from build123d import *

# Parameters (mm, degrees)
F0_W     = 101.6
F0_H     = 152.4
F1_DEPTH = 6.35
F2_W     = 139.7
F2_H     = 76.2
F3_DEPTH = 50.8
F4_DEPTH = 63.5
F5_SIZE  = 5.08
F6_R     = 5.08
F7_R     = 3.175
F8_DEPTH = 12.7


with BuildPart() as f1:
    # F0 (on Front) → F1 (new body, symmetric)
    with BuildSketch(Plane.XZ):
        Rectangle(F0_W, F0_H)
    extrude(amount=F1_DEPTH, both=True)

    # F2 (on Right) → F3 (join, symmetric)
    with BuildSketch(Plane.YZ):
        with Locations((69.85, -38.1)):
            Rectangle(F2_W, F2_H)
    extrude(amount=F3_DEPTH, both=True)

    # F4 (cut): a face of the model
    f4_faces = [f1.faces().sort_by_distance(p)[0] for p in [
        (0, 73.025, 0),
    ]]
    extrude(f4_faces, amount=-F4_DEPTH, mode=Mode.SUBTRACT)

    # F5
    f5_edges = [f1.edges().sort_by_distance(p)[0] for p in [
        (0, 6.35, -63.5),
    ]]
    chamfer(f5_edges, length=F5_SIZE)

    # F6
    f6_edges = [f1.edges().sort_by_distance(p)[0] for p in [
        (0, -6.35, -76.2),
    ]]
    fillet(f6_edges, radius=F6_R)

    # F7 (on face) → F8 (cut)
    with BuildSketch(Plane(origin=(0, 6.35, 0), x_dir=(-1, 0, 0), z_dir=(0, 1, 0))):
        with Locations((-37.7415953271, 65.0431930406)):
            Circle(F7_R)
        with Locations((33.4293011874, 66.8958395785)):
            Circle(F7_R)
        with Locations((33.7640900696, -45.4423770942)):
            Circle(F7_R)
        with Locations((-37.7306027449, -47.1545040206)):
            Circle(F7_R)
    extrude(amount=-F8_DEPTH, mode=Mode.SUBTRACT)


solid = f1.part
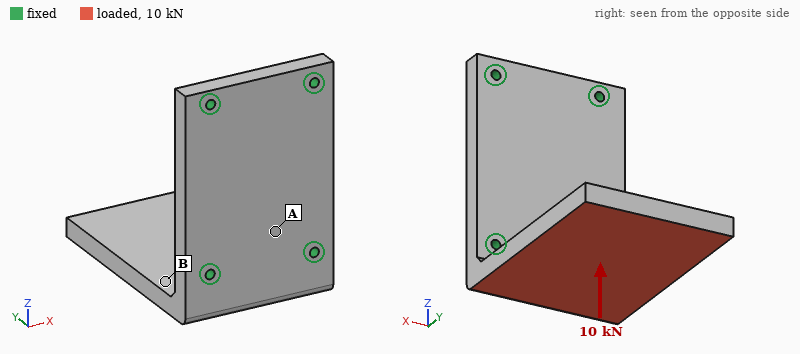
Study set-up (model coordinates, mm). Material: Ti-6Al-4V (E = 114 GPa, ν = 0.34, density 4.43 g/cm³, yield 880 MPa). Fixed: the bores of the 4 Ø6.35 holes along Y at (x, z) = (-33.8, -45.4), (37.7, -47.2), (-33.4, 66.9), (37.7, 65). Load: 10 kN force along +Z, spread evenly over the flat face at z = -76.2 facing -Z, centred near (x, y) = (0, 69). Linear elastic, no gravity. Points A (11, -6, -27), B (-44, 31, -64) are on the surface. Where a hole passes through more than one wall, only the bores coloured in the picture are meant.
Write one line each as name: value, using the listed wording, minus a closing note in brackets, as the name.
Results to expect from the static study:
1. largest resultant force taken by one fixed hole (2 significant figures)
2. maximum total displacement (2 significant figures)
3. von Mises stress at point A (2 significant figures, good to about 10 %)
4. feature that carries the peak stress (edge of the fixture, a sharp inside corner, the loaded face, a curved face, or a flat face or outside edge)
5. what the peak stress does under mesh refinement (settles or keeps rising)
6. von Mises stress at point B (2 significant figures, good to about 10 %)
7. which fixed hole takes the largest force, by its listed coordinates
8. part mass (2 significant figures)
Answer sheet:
largest resultant force taken by one fixed hole: 4.7 kN
maximum total displacement: 2.5 mm
von Mises stress at point A: 52 MPa
feature that carries the peak stress: edge of the fixture
what the peak stress does under mesh refinement: keeps rising
von Mises stress at point B: 140 MPa
which fixed hole takes the largest force, by its listed coordinates: (-33.8, -45.4)
part mass: 1.6 kg
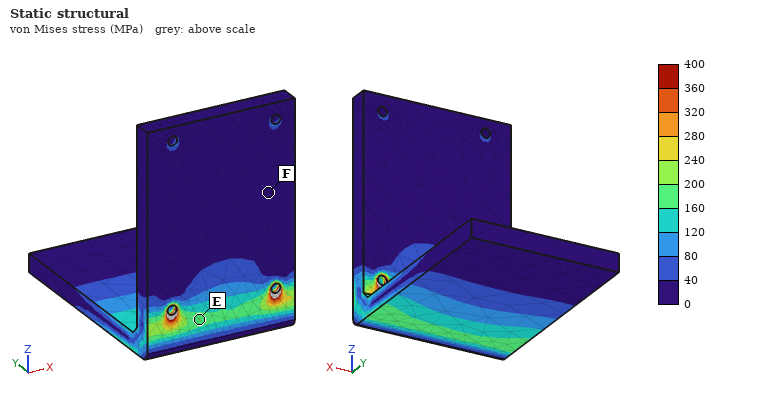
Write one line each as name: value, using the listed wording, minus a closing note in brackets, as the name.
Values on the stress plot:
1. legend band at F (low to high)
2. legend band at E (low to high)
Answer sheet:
legend band at F: 0 to 40 MPa
legend band at E: 160 to 200 MPa
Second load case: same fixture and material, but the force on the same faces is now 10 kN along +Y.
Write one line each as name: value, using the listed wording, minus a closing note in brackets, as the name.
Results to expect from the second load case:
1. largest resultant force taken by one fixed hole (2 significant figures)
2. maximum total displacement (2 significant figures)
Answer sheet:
largest resultant force taken by one fixed hole: 5.5 kN
maximum total displacement: 0.55 mm
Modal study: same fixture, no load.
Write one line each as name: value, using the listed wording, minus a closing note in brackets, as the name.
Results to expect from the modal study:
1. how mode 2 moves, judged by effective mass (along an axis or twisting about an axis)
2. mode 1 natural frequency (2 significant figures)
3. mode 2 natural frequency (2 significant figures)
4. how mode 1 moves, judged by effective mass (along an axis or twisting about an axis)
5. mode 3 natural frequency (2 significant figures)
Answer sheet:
how mode 2 moves, judged by effective mass: along X
mode 1 natural frequency: 440 Hz
mode 2 natural frequency: 1300 Hz
how mode 1 moves, judged by effective mass: along Z
mode 3 natural frequency: 1800 Hz
